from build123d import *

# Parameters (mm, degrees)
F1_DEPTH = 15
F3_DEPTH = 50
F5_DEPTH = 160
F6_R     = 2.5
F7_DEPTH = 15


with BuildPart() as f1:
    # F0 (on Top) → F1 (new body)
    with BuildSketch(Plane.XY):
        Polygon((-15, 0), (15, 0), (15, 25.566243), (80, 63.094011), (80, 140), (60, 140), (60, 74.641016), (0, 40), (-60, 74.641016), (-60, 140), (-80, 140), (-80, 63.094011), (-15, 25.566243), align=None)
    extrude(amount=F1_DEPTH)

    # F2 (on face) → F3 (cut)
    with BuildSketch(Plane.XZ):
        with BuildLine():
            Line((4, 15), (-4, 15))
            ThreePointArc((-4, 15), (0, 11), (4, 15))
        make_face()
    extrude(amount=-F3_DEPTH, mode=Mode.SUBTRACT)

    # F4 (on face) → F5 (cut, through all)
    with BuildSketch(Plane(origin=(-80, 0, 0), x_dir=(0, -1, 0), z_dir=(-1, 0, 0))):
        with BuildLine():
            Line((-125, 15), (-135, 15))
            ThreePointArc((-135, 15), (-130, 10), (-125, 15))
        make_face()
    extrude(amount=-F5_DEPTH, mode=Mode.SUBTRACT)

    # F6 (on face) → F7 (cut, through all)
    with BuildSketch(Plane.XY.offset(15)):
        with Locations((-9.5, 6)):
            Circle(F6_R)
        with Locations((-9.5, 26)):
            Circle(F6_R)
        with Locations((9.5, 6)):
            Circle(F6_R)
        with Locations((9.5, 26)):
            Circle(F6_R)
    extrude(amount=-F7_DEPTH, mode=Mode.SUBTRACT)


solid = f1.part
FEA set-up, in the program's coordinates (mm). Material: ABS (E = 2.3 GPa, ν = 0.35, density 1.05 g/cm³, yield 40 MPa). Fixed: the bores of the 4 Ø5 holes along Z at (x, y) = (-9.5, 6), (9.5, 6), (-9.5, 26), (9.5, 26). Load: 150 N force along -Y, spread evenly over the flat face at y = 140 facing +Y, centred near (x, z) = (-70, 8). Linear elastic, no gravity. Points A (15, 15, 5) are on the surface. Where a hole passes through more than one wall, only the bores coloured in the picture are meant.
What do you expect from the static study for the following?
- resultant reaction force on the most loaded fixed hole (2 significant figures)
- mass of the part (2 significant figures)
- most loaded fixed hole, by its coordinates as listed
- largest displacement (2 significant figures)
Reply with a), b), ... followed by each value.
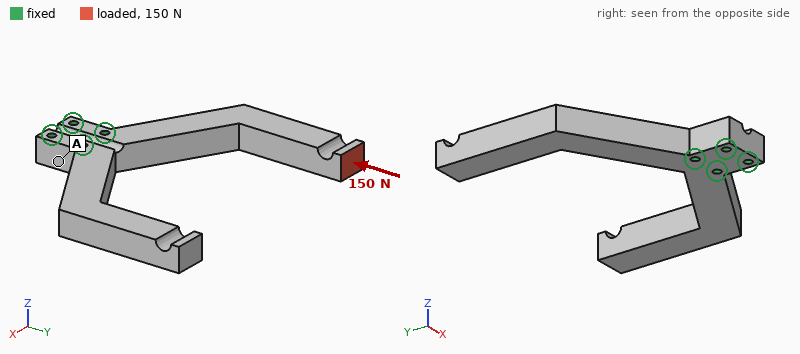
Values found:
a) 530 N
b) 100 g
c) (-9.5, 26)
d) 1.9 mm
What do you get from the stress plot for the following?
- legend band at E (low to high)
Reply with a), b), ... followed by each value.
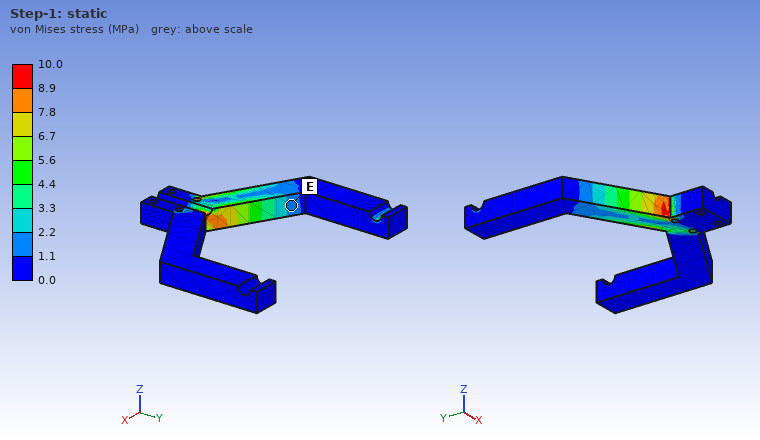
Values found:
a) 1.1 to 2.2 MPa
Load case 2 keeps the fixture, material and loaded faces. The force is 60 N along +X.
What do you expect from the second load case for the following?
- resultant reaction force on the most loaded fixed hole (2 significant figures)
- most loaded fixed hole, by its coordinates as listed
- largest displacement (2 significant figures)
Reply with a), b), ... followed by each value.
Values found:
a) 340 N
b) (9.5, 26)
c) 2.2 mm
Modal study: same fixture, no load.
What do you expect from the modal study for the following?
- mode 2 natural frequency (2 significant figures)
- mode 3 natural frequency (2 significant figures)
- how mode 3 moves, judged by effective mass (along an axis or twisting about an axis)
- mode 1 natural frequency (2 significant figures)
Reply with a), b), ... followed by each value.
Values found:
a) 190 Hz
b) 240 Hz
c) along X
d) 190 Hz
